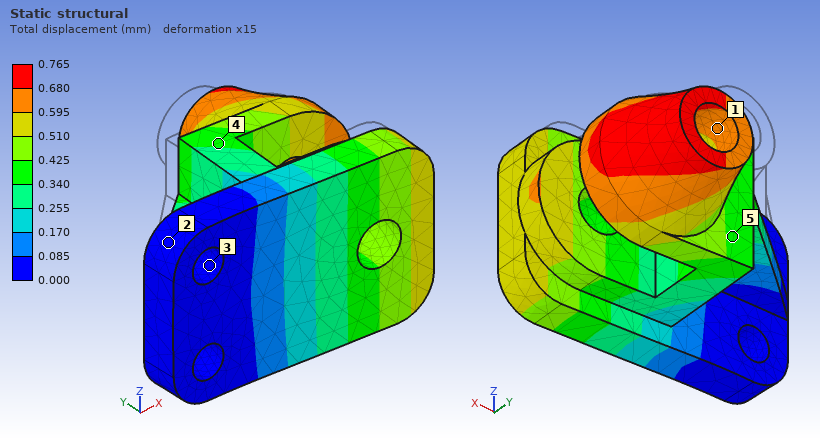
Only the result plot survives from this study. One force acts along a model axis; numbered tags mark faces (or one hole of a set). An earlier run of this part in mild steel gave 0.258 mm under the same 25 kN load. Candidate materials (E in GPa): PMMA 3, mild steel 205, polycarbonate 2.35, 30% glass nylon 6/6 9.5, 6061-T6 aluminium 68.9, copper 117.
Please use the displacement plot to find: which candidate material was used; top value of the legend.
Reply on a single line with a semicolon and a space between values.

6061-T6 aluminium; 0.765 mm
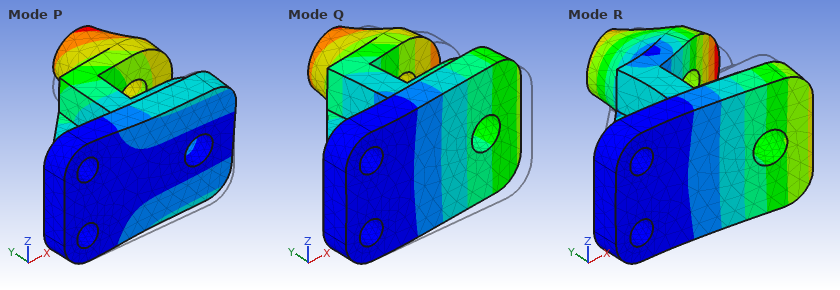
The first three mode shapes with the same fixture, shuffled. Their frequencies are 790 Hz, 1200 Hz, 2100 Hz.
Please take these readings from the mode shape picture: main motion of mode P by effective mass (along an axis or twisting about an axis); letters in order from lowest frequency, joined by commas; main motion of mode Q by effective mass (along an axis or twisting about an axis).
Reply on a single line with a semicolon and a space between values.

along Z; Q, P, R; along Y
